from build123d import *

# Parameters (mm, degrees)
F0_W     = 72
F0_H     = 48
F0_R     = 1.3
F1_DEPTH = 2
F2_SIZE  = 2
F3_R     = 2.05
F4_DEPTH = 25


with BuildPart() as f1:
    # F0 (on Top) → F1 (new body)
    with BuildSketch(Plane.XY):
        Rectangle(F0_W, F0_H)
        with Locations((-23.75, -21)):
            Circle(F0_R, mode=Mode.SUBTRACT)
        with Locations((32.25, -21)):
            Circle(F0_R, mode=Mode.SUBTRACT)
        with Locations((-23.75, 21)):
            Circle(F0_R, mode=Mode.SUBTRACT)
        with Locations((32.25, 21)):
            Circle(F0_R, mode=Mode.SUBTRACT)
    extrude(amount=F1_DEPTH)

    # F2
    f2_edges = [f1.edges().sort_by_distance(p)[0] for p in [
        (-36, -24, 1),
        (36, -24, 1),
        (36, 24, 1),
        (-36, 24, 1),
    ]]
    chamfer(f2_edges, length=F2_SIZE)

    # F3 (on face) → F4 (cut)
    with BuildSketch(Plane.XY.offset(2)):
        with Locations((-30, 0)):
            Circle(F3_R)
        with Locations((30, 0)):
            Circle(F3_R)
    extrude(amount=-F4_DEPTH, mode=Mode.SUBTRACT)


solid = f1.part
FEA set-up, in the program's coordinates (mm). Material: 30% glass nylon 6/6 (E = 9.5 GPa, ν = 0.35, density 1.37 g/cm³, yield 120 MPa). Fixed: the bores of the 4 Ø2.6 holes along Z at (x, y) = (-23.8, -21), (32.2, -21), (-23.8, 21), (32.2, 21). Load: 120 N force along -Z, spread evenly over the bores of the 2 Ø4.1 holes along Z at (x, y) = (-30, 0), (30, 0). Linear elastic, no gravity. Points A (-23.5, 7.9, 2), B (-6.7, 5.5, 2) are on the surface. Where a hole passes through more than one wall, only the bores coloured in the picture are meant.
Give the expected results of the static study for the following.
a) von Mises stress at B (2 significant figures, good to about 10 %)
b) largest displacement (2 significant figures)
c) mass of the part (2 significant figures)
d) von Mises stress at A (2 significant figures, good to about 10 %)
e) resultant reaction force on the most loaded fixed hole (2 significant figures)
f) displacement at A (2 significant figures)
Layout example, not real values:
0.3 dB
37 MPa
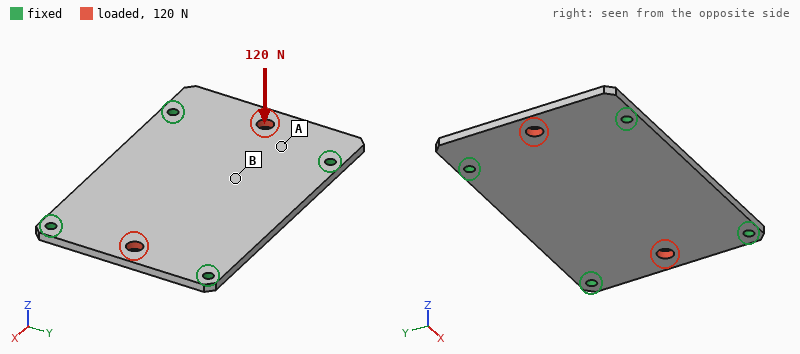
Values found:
5.5 MPa
0.38 mm
9.3 g
12 MPa
32 N
0.14 mm
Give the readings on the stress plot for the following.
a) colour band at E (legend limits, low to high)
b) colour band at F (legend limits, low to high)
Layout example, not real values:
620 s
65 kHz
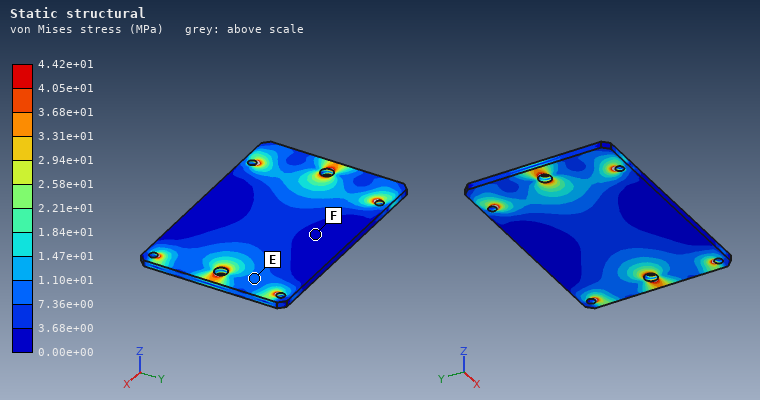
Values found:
7.36e+00 to 1.10e+01 MPa
0.00e+00 to 3.68e+00 MPa
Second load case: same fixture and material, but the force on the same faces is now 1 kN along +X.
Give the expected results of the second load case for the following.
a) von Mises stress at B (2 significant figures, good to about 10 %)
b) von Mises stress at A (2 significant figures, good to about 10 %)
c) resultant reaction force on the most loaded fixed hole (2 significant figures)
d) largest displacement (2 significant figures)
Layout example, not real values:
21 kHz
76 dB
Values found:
4.7 MPa
9.3 MPa
280 N
58 µm
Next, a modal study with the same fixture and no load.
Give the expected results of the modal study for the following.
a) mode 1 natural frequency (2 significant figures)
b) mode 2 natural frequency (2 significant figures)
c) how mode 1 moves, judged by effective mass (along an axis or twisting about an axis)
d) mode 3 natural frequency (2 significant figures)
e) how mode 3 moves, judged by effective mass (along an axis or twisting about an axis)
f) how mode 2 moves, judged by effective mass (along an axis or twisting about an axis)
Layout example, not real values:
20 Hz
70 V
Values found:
1400 Hz
2200 Hz
along Z
2600 Hz
along Z
twisting about X
